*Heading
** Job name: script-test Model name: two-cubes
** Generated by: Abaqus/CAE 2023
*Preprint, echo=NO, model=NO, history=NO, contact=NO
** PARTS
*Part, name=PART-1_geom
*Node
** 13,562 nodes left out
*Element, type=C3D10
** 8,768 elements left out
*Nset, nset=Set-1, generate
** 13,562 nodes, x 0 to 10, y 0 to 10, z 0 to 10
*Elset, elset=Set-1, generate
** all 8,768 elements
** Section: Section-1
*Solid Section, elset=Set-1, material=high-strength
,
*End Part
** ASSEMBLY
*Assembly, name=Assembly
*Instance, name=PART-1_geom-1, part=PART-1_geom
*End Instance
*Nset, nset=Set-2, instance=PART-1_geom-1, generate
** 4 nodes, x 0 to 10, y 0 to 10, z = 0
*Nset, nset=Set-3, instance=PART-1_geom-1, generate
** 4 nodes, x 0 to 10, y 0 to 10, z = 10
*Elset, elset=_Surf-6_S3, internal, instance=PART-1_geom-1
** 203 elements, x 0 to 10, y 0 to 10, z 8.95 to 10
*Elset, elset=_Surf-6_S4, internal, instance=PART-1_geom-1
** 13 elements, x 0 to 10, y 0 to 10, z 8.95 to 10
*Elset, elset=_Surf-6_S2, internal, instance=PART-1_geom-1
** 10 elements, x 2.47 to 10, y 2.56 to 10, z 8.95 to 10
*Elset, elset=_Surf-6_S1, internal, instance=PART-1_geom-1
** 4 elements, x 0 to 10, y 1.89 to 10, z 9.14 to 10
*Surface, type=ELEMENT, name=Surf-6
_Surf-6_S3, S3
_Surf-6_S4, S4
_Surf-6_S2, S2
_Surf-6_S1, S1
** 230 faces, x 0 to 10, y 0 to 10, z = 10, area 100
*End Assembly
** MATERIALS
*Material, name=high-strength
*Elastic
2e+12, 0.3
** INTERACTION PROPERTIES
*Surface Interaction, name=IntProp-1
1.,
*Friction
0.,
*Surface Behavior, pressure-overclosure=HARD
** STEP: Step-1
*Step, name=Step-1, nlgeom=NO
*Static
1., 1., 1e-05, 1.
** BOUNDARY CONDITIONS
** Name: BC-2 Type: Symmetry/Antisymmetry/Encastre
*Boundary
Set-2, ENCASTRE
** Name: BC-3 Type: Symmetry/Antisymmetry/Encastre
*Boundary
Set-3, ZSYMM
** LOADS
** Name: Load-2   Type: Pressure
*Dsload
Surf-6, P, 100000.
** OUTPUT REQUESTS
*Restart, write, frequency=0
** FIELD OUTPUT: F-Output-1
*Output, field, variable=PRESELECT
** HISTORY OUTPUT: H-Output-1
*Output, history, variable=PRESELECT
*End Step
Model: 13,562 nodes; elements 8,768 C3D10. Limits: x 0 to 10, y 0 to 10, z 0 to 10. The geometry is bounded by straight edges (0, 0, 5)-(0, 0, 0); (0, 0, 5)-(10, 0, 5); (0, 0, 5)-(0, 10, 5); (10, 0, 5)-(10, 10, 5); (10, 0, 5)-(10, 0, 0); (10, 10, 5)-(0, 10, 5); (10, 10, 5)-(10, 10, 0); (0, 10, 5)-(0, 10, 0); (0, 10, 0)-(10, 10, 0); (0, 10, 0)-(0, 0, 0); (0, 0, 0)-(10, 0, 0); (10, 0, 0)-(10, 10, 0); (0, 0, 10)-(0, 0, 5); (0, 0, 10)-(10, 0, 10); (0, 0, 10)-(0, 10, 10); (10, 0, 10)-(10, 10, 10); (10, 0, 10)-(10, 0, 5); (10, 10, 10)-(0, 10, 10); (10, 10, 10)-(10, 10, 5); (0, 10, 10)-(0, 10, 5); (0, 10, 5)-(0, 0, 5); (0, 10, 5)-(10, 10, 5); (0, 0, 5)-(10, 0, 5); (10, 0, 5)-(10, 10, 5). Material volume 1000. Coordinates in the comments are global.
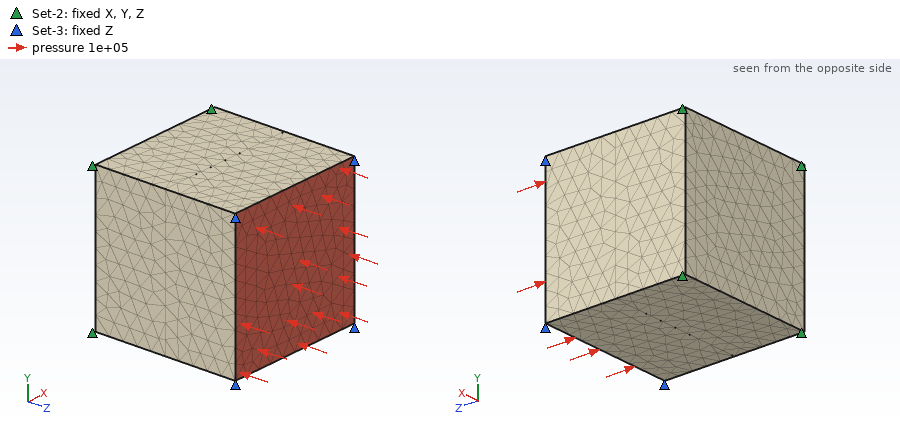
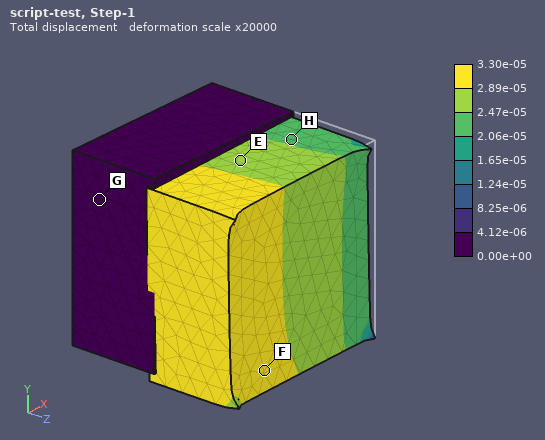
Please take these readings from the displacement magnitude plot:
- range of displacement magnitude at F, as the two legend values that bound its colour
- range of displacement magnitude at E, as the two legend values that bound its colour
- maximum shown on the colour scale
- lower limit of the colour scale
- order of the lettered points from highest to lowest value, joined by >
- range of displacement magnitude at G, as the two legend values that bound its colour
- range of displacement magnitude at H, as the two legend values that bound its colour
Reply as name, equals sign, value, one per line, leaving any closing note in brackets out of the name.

range of displacement magnitude at F, as the two legend values that bound its colour = 2.89e-05 to 3.30e-05
range of displacement magnitude at E, as the two legend values that bound its colour = 2.47e-05 to 2.89e-05
maximum shown on the colour scale = 3.30e-05
lower limit of the colour scale = 0.00e+00
order of the lettered points from highest to lowest value, joined by > = F > E > H > G
range of displacement magnitude at G, as the two legend values that bound its colour = 0.00e+00 to 4.12e-06
range of displacement magnitude at H, as the two legend values that bound its colour = 2.06e-05 to 2.47e-05
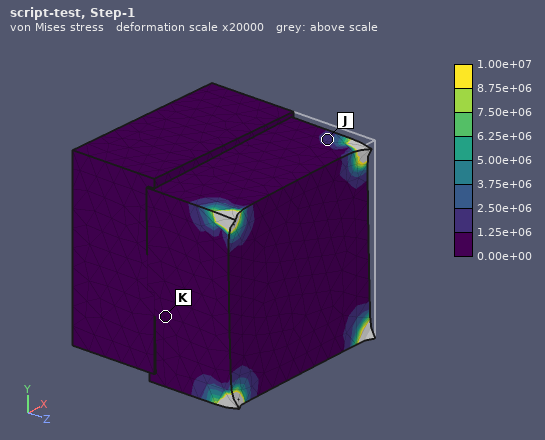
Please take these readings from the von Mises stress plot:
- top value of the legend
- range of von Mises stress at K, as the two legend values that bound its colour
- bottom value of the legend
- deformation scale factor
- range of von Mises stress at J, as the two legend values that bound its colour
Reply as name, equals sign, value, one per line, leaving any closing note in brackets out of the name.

top value of the legend = 1.00e+07
range of von Mises stress at K, as the two legend values that bound its colour = 0.00e+00 to 1.25e+06
bottom value of the legend = 0.00e+00
deformation scale factor = 20000
range of von Mises stress at J, as the two legend values that bound its colour = 1.25e+06 to 2.50e+06
